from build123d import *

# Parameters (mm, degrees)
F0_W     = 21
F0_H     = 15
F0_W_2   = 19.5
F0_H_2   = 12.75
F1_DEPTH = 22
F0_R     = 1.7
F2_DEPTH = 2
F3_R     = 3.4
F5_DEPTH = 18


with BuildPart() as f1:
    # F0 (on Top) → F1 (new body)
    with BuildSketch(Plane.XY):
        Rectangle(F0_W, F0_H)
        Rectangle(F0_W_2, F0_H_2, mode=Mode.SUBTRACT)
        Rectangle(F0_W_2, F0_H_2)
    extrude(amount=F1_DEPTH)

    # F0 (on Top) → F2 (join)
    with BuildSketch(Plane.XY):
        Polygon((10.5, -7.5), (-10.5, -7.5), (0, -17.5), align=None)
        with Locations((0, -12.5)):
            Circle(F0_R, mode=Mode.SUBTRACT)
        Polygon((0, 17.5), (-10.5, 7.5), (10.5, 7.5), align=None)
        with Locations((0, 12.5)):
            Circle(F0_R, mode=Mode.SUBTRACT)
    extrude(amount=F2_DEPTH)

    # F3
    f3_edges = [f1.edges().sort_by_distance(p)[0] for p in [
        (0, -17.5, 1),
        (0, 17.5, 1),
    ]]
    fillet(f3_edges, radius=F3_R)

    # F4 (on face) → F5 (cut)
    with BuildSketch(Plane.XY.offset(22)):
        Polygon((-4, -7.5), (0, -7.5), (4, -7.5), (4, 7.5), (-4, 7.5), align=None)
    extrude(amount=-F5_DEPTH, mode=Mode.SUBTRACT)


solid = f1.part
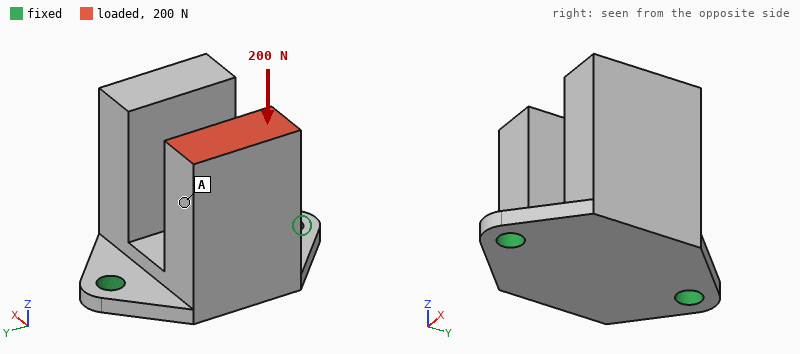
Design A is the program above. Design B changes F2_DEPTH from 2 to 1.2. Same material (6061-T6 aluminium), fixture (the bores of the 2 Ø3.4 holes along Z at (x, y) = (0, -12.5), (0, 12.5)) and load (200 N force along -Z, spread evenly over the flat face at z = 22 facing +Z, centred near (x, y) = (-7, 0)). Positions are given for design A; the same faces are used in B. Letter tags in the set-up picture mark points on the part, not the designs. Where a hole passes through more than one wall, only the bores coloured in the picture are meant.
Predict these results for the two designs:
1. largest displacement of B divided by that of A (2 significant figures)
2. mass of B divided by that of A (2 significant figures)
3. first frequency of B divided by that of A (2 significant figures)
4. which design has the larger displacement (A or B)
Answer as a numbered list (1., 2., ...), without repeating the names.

1. 3.2
2. 0.97
3. 0.55
4. B
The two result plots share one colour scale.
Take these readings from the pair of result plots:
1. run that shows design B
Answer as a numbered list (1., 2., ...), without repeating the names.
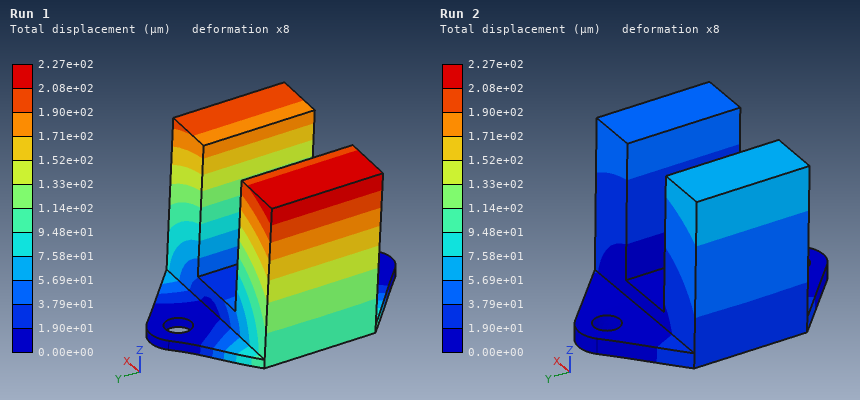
1. Run 1
